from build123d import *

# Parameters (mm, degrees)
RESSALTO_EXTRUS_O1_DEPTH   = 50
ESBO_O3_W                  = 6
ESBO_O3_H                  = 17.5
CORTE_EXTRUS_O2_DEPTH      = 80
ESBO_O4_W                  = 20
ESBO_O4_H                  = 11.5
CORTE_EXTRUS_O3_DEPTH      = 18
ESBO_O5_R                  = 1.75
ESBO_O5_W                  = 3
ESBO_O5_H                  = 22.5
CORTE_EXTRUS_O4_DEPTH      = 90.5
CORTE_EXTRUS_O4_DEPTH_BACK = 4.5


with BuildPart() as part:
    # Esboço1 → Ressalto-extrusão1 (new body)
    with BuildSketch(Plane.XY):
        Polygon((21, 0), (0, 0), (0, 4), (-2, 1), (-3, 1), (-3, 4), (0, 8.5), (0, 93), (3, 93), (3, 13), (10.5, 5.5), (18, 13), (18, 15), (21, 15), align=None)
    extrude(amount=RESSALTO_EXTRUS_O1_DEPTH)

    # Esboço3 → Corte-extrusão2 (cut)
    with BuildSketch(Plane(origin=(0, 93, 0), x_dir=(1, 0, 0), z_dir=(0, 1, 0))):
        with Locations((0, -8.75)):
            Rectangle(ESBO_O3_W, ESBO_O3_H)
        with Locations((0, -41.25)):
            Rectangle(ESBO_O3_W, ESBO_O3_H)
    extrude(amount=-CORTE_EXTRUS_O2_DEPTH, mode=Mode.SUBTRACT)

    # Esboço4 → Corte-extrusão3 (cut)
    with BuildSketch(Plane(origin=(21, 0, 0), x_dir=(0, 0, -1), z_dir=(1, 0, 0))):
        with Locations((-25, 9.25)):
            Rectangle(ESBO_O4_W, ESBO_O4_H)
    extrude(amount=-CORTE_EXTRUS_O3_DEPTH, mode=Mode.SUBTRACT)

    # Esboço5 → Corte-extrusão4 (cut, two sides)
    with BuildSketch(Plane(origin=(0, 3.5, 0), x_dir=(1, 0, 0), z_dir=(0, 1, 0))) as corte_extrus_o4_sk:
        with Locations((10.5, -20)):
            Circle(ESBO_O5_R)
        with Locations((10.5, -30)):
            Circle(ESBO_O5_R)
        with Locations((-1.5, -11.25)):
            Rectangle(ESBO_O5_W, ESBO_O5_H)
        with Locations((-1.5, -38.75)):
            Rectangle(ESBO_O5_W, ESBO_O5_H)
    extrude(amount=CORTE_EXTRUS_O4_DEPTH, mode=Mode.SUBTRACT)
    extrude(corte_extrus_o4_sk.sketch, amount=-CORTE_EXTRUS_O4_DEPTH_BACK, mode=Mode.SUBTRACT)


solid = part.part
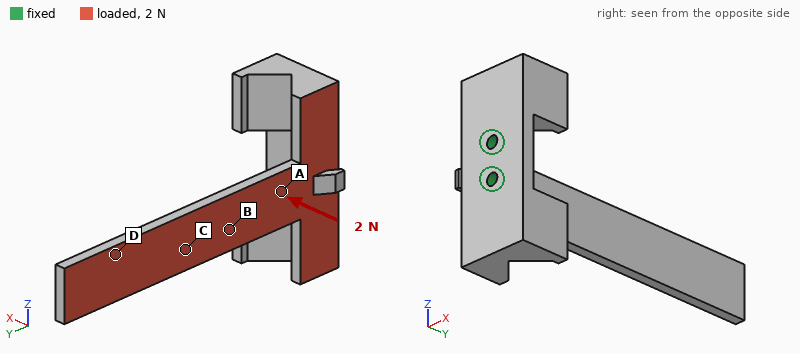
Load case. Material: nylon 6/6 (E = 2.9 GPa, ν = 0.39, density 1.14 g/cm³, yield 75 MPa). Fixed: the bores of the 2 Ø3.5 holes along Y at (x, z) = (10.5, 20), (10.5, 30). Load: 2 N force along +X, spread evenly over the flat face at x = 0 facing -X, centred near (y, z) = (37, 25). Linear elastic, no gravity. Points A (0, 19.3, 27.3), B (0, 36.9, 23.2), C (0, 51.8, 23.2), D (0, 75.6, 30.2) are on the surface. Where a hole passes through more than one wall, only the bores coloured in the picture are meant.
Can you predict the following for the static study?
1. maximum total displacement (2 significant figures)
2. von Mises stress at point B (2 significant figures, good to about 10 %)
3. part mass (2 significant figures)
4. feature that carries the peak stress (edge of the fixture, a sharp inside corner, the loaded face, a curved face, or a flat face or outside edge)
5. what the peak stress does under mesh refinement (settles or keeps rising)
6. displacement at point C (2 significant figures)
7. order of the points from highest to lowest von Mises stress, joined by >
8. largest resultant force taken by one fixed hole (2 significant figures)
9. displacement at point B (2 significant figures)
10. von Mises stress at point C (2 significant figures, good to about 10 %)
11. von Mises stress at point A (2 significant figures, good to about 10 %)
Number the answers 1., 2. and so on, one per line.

1. 1.2 mm
2. 1.2 MPa
3. 14 g
4. a sharp inside corner
5. keeps rising
6. 0.44 mm
7. A > B > C > D
8. 1.0 N
9. 0.23 mm
10. 0.62 MPa
11. 2.0 MPa
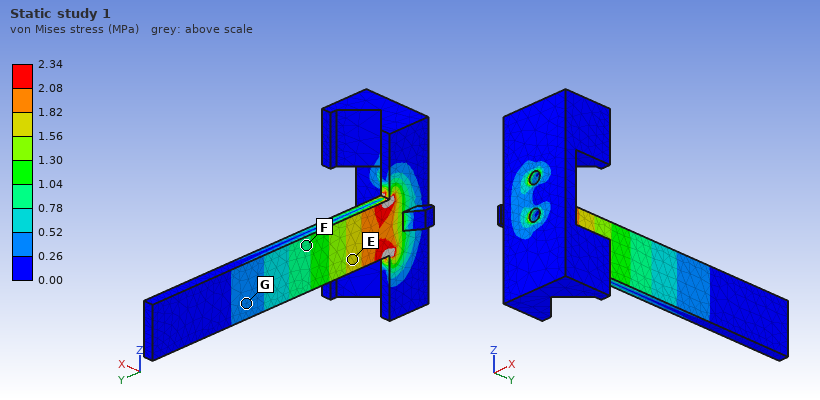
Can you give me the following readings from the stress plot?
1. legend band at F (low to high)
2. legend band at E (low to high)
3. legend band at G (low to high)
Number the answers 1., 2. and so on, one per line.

1. 0.78 to 1.04 MPa
2. 1.56 to 1.82 MPa
3. 0.26 to 0.52 MPa
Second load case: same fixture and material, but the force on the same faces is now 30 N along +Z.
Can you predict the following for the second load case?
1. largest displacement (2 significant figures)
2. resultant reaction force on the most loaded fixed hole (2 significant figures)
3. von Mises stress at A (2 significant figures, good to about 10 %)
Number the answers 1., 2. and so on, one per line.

1. 1.2 mm
2. 68 N
3. 2.3 MPa
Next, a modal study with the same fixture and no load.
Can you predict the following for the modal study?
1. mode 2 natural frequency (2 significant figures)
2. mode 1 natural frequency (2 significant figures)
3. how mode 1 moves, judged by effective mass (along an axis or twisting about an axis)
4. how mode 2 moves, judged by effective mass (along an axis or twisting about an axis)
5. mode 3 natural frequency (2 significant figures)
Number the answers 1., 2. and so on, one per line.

1. 390 Hz
2. 100 Hz
3. along X
4. along Z
5. 640 Hz
